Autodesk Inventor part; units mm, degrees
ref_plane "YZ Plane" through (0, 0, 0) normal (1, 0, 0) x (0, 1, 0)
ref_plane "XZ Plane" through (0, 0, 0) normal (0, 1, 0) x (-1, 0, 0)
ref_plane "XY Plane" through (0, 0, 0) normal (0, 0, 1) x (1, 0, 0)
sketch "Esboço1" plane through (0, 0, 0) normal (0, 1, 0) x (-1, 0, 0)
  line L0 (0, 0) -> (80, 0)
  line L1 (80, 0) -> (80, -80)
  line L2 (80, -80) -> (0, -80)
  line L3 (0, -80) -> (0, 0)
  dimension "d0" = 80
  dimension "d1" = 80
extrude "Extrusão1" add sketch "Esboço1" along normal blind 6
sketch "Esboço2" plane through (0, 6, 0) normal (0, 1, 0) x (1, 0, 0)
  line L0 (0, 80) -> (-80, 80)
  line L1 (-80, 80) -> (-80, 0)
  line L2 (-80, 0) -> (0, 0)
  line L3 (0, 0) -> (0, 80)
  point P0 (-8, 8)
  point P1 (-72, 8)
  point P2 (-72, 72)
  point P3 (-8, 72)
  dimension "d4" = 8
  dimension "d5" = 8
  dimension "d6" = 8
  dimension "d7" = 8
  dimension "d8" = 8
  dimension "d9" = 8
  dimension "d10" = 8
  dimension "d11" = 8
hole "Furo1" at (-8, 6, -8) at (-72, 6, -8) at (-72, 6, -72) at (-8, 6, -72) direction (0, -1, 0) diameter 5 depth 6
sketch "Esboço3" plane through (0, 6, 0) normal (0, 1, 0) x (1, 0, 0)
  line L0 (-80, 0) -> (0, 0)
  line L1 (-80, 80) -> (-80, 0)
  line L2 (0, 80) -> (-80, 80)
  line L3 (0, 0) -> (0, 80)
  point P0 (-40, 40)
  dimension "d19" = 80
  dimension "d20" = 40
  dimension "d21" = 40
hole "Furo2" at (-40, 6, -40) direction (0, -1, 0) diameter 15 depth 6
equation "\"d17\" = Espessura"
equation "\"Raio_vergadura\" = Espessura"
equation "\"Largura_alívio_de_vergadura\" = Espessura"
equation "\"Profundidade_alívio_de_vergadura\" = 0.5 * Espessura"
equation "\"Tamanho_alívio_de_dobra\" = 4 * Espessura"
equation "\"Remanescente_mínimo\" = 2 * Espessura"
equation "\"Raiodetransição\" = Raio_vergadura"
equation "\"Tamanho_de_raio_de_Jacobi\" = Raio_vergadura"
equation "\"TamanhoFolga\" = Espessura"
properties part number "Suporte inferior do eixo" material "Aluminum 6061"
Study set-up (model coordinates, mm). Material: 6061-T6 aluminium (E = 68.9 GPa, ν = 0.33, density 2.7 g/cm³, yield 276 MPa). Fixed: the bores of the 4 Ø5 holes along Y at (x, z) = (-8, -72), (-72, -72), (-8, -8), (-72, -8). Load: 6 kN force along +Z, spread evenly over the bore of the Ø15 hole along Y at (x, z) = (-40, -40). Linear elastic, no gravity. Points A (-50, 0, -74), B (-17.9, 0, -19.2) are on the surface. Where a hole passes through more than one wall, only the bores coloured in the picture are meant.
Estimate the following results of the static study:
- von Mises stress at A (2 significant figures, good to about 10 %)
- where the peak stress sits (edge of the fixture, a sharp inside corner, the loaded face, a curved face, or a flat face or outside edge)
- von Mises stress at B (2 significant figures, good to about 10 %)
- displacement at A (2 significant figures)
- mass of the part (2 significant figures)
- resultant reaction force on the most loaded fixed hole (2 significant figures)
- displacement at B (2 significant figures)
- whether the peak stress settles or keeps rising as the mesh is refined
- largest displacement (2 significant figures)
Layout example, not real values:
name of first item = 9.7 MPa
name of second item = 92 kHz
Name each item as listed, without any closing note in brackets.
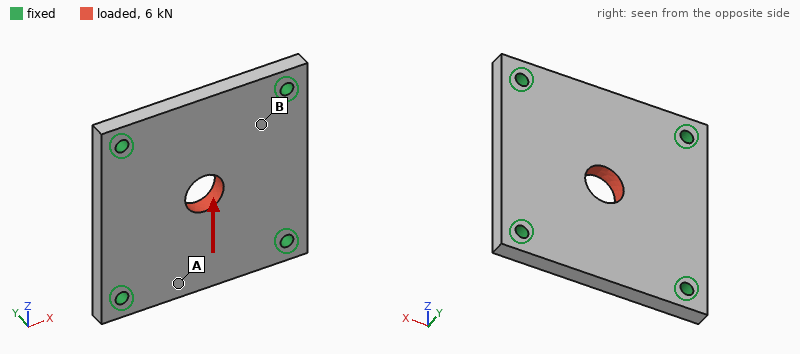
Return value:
von Mises stress at A = 5.5 MPa
where the peak stress sits = edge of the fixture
von Mises stress at B = 15 MPa
displacement at A = 7.1 µm
mass of the part = 100 g
resultant reaction force on the most loaded fixed hole = 1.7 kN
displacement at B = 4.2 µm
whether the peak stress settles or keeps rising as the mesh is refined = keeps rising
largest displacement = 12 µm
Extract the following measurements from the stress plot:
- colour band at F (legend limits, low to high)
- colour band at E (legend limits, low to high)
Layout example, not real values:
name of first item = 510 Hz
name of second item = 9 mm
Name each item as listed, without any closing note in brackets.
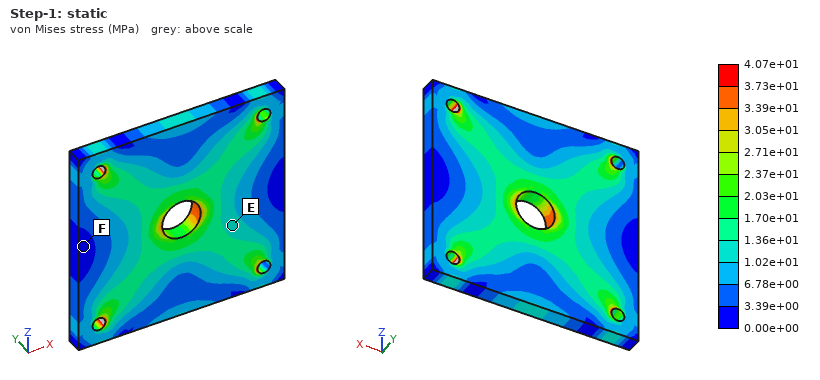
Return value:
colour band at F = 0.00e+00 to 3.39e+00 MPa
colour band at E = 1.02e+01 to 1.36e+01 MPa
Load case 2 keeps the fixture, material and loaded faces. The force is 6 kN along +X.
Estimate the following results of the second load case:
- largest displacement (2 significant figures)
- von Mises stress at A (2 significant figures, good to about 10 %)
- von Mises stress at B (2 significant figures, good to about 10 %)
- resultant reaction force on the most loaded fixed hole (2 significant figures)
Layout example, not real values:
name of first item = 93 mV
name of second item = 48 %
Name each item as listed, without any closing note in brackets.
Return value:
largest displacement = 12 µm
von Mises stress at A = 4.8 MPa
von Mises stress at B = 15 MPa
resultant reaction force on the most loaded fixed hole = 1.7 kN
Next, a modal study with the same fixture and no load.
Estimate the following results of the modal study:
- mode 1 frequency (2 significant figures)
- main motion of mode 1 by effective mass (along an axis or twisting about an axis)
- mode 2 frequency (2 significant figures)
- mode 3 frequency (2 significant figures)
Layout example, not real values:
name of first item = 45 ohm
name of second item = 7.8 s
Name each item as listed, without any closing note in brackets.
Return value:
mode 1 frequency = 5000 Hz
main motion of mode 1 by effective mass = along Y
mode 2 frequency = 8000 Hz
mode 3 frequency = 8000 Hz
